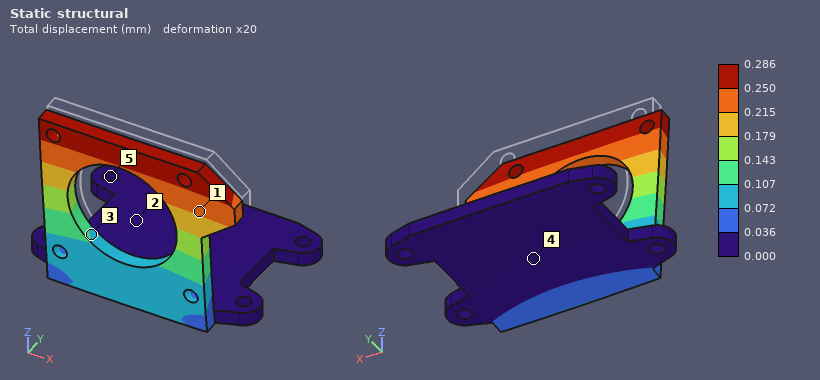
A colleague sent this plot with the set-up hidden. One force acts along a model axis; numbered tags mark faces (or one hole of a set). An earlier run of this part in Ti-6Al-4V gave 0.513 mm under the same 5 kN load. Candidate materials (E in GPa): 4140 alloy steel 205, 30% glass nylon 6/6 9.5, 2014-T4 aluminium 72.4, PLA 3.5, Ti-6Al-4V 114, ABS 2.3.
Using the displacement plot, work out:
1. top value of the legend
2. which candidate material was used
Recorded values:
0.286 mm
4140 alloy steel
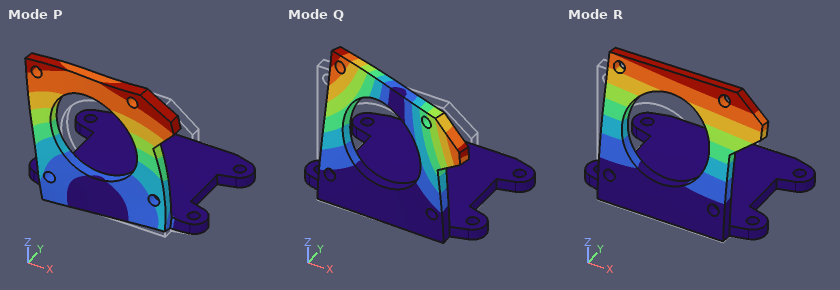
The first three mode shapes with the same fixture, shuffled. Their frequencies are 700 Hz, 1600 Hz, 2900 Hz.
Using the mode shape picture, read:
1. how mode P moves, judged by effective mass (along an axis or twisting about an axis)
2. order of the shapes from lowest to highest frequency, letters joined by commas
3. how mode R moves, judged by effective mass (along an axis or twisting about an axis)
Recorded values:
along X
R, Q, P
along Y
